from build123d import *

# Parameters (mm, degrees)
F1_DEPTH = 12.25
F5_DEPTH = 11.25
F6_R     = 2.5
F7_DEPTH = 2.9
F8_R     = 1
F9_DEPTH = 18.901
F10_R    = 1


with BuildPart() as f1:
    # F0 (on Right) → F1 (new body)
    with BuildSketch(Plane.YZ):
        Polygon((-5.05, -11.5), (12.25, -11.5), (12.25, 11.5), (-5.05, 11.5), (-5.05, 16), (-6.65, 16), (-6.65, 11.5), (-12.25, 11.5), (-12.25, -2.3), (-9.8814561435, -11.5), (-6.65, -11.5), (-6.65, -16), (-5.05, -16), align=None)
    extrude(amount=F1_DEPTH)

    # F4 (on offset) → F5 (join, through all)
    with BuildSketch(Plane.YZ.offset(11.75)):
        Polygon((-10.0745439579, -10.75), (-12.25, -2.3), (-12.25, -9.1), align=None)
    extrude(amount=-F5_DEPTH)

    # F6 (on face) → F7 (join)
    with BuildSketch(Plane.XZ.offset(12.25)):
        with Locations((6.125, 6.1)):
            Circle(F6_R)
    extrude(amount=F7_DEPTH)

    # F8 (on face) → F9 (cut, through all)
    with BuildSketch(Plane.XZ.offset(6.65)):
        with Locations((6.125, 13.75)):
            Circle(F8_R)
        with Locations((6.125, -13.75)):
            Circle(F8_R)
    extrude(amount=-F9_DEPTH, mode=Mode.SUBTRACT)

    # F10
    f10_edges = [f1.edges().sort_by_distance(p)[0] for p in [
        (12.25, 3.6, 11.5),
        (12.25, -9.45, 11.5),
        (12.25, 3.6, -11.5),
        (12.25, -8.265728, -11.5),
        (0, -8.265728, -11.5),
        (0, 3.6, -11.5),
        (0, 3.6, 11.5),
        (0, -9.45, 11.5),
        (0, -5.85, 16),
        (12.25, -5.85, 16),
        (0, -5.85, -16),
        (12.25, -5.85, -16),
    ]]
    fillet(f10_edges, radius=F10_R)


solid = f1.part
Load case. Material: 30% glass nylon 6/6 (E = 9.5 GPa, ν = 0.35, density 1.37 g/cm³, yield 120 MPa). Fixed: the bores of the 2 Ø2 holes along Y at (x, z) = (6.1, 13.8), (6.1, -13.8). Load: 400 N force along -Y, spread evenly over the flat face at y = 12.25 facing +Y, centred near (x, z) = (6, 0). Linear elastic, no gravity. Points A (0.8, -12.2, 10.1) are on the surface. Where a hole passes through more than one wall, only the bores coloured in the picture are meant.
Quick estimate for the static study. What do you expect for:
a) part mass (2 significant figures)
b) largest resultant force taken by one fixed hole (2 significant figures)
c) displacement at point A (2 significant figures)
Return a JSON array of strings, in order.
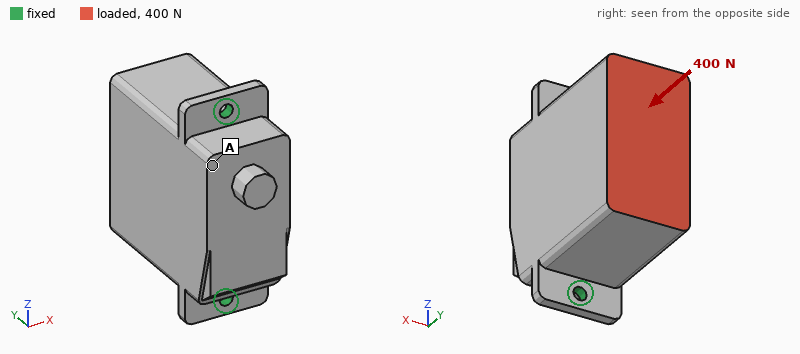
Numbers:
["9.7 g", "200 N", "24 µm"]
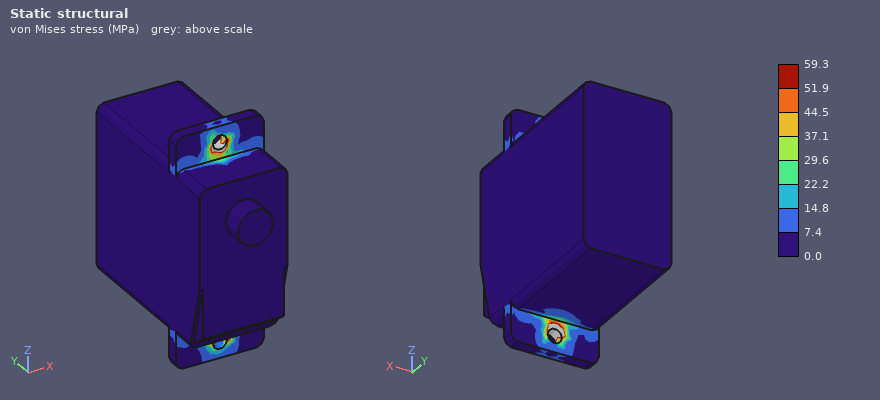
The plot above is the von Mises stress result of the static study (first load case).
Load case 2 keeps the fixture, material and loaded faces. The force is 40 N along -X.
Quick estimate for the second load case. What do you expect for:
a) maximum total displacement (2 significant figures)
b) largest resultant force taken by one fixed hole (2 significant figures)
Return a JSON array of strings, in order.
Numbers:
["0.25 mm", "20 N"]
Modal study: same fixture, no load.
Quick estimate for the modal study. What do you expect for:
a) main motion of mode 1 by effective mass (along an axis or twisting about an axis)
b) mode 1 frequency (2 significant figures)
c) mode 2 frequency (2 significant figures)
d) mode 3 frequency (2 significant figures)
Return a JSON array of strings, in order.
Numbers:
["along X", "1200 Hz", "6400 Hz", "6500 Hz"]
